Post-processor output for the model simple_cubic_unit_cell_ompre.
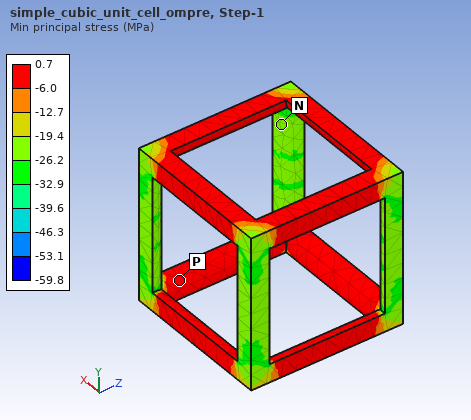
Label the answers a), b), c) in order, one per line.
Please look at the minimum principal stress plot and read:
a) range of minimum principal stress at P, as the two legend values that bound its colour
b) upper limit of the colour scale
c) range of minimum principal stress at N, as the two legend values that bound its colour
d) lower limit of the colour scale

a) -6.0 to 0.7 MPa
b) 0.7 MPa
c) -26.2 to -19.4 MPa
d) -59.8 MPa
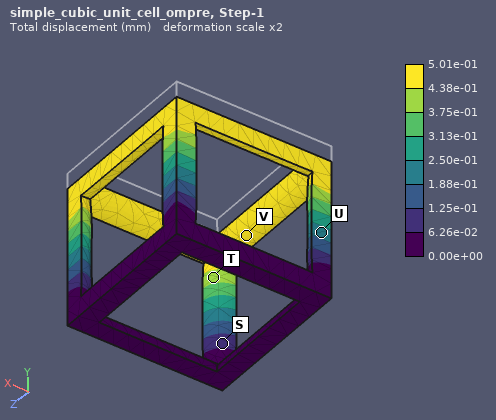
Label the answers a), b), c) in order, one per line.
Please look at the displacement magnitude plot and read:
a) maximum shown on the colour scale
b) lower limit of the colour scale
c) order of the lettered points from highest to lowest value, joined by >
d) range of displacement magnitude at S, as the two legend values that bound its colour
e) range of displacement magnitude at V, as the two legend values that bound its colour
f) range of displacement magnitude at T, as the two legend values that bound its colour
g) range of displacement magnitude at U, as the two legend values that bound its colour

a) 5.01e-01 mm
b) 0.00e+00 mm
c) V > T > U > S
d) 6.26e-02 to 1.25e-01 mm
e) 4.38e-01 to 5.01e-01 mm
f) 3.75e-01 to 4.38e-01 mm
g) 1.88e-01 to 2.50e-01 mm
